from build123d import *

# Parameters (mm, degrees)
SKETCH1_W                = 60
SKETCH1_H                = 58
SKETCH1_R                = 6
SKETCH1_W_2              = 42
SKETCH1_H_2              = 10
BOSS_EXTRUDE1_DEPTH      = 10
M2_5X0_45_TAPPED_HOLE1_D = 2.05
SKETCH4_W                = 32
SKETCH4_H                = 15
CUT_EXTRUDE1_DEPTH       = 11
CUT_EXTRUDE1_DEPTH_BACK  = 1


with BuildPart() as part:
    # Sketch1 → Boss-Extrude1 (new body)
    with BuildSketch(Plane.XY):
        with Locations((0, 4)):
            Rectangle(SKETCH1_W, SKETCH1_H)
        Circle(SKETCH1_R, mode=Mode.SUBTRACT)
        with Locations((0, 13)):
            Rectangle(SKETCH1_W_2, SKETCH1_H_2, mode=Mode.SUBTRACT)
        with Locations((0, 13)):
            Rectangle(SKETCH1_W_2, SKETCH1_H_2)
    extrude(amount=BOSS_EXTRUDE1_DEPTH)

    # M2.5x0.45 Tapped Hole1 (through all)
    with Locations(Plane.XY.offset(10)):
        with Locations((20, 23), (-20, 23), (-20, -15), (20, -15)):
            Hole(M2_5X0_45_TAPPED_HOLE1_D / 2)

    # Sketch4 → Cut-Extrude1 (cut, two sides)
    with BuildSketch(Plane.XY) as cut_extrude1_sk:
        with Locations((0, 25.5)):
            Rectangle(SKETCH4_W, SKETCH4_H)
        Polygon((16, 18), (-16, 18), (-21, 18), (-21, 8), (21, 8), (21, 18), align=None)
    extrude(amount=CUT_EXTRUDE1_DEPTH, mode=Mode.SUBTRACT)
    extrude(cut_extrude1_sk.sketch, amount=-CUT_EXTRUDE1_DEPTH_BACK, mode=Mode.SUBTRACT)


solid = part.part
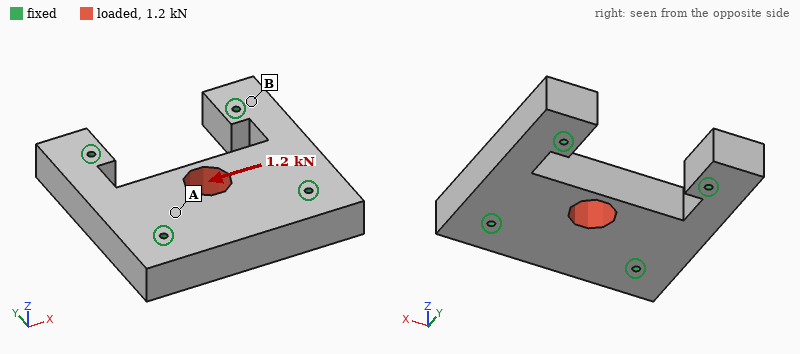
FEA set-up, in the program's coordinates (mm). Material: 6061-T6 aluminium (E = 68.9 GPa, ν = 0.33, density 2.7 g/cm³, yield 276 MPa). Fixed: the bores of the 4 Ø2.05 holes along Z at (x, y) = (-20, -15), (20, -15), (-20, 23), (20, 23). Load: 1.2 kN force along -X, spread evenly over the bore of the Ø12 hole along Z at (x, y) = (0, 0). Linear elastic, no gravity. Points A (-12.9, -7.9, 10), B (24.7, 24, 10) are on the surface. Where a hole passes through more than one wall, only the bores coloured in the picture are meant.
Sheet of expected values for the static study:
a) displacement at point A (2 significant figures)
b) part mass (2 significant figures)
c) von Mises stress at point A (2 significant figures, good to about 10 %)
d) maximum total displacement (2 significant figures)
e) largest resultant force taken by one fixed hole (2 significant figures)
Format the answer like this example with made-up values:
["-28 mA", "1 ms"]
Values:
["0.91 µm", "66 g", "3.4 MPa", "2.7 µm", "550 N"]
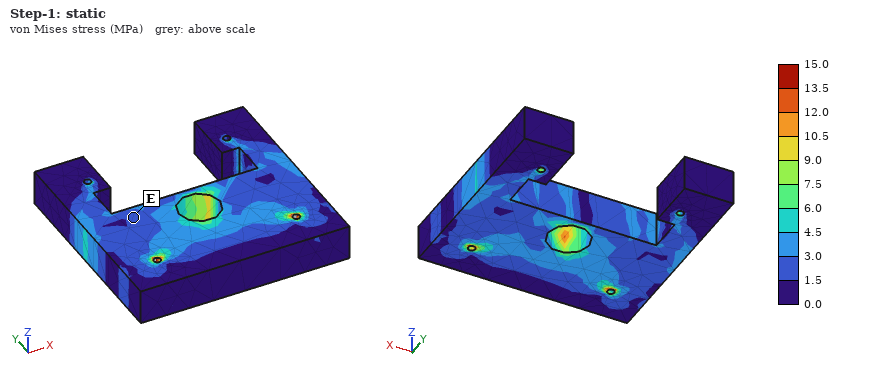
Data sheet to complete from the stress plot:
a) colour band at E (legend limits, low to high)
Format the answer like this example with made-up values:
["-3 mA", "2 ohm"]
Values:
["1.5 to 3.0 MPa"]
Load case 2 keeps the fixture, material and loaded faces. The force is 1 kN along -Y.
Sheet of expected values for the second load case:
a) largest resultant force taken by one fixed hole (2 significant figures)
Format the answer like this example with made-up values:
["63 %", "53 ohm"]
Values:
["520 N"]
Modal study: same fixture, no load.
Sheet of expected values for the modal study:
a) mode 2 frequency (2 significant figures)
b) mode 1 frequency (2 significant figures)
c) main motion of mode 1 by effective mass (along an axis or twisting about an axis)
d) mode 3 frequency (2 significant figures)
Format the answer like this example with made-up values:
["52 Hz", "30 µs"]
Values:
["19 kHz", "13 kHz", "along Z", "20 kHz"]
